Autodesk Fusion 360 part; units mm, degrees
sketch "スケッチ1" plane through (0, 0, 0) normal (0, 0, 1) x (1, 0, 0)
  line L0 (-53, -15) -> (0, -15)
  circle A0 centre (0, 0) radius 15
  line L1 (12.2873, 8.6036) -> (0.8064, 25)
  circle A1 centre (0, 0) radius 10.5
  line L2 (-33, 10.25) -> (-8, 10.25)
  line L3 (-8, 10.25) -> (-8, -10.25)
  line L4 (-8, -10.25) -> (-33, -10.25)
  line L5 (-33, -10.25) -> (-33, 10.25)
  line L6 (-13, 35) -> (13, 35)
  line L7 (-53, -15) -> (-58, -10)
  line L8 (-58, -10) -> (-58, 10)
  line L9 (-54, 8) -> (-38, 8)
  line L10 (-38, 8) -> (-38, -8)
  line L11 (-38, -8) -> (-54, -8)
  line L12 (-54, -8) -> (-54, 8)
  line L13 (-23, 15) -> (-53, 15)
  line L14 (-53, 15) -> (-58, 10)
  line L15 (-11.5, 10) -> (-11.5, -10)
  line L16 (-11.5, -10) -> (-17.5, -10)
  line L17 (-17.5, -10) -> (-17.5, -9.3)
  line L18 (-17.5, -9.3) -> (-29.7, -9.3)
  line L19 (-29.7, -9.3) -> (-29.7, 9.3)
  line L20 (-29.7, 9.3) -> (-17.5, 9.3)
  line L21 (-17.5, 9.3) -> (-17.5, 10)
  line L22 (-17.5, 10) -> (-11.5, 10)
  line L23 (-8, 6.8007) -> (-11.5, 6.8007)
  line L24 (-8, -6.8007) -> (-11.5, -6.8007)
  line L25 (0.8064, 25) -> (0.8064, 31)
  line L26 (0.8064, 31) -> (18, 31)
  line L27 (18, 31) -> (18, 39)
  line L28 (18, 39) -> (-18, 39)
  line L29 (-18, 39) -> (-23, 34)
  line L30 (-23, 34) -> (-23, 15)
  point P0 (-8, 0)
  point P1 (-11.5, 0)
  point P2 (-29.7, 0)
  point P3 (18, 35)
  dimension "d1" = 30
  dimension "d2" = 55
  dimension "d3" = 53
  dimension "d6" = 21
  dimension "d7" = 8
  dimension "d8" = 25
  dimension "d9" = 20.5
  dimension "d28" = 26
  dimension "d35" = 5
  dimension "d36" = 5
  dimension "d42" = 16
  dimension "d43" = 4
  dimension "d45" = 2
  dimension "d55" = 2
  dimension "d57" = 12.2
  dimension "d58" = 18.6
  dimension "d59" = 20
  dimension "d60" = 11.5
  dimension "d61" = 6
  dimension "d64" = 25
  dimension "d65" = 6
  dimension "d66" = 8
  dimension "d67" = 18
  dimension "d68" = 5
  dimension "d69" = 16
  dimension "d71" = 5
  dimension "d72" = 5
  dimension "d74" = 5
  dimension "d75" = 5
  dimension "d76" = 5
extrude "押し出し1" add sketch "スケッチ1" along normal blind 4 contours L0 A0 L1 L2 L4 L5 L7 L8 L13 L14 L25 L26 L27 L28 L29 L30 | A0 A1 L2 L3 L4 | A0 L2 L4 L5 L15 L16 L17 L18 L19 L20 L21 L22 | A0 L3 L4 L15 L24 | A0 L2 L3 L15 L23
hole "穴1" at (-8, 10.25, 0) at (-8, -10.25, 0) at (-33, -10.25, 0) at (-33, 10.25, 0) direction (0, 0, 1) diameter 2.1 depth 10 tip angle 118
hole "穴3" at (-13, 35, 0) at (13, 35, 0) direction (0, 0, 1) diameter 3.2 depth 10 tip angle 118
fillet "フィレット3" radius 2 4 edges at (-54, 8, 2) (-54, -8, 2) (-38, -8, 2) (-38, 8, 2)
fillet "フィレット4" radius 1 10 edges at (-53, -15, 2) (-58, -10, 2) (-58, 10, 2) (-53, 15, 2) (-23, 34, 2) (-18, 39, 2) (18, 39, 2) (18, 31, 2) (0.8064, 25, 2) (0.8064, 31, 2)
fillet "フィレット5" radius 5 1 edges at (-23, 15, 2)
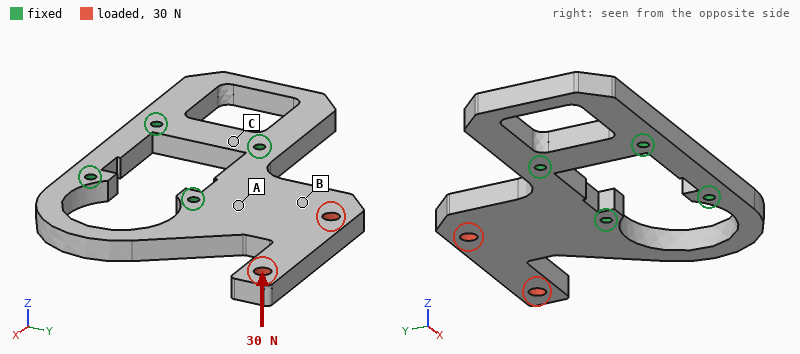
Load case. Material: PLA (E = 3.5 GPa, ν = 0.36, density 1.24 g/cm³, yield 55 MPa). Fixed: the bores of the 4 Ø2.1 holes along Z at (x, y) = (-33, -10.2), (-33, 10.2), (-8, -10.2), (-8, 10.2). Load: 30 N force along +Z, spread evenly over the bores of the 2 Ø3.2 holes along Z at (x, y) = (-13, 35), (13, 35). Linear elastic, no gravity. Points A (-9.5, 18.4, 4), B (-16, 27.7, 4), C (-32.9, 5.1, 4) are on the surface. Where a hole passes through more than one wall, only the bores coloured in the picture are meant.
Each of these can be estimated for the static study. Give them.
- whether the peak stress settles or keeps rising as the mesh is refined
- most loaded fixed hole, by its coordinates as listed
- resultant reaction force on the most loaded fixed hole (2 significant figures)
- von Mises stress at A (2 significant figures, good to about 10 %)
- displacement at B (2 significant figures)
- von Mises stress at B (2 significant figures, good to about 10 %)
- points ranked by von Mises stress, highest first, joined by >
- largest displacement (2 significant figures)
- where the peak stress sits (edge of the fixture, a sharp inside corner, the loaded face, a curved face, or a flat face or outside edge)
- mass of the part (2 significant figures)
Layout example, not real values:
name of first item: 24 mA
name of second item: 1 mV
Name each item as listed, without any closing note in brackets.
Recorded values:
whether the peak stress settles or keeps rising as the mesh is refined: keeps rising
most loaded fixed hole, by its coordinates as listed: (-8, 10.2)
resultant reaction force on the most loaded fixed hole: 42 N
von Mises stress at A: 7.5 MPa
displacement at B: 0.24 mm
von Mises stress at B: 4.1 MPa
points ranked by von Mises stress, highest first, joined by >: A > B > C
largest displacement: 1.1 mm
where the peak stress sits: edge of the fixture
mass of the part: 9.0 g
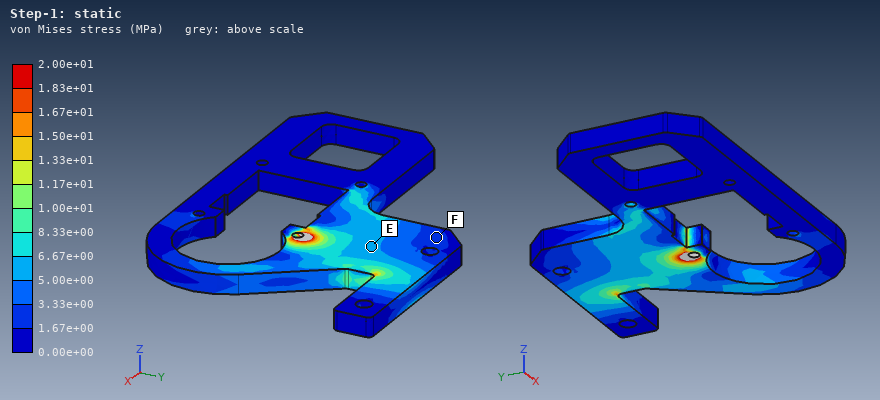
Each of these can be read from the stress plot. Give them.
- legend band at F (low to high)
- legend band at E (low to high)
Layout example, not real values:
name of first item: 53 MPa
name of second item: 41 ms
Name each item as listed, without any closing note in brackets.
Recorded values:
legend band at F: 1.67e+00 to 3.33e+00 MPa
legend band at E: 5.00e+00 to 6.67e+00 MPa
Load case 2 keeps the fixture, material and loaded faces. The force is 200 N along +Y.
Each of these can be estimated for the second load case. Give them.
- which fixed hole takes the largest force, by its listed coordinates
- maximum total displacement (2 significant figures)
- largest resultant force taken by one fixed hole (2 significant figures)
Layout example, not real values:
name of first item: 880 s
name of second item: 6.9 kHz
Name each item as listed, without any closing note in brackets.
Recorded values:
which fixed hole takes the largest force, by its listed coordinates: (-8, 10.2)
maximum total displacement: 0.59 mm
largest resultant force taken by one fixed hole: 250 N
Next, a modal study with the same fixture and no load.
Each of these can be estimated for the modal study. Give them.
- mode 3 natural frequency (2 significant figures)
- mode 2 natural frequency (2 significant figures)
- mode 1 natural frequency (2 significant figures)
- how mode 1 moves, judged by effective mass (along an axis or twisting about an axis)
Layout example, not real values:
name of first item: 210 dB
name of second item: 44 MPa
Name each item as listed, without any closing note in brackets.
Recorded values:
mode 3 natural frequency: 1500 Hz
mode 2 natural frequency: 1500 Hz
mode 1 natural frequency: 860 Hz
how mode 1 moves, judged by effective mass: along Z
